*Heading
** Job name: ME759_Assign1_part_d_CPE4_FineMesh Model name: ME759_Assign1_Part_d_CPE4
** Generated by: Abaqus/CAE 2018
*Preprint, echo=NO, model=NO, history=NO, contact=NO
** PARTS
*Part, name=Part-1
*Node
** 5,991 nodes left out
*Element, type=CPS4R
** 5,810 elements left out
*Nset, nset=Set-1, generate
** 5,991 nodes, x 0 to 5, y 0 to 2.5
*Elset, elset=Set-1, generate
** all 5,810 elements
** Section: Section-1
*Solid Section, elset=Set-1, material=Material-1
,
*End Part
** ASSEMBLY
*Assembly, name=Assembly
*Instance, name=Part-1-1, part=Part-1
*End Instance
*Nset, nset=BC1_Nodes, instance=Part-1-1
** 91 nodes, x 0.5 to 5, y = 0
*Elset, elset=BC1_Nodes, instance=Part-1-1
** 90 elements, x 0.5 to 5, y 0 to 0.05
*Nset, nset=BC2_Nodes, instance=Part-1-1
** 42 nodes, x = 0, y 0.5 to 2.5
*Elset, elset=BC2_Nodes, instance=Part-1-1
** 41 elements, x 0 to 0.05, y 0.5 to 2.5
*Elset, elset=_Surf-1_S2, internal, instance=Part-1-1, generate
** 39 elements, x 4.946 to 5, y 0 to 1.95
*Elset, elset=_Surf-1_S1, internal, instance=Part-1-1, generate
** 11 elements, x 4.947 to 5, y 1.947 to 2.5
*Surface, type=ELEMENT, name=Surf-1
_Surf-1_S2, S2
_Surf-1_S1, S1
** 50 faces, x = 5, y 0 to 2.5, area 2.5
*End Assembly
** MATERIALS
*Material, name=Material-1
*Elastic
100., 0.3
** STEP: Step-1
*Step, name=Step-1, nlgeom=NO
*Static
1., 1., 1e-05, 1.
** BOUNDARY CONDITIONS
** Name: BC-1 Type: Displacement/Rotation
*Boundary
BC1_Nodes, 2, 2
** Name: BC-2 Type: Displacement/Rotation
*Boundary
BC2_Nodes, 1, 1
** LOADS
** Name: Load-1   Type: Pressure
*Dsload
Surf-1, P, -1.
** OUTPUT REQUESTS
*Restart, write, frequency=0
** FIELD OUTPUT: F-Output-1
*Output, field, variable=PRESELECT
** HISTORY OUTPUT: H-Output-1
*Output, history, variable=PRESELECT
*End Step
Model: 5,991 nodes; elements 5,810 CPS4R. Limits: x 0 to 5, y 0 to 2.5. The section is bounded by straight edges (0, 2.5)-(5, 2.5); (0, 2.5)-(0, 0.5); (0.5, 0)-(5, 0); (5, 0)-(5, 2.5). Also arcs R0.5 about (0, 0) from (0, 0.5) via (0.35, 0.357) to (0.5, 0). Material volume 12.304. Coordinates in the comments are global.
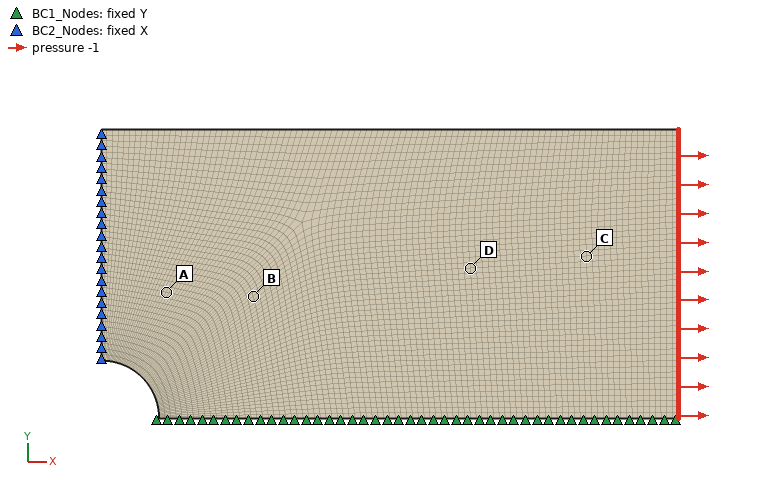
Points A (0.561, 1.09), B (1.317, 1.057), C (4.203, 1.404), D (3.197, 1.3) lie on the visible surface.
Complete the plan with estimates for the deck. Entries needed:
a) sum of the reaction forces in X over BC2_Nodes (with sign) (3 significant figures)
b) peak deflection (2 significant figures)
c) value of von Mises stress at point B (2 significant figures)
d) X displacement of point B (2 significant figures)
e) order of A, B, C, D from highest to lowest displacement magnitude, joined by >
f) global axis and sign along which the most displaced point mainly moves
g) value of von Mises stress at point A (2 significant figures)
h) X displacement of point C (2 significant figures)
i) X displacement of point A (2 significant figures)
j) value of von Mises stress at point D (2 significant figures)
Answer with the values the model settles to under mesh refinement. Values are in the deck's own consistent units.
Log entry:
-2.50
0.053
1.1
0.016
C > D > B > A
+X
1.2
0.044
0.0066
1.0
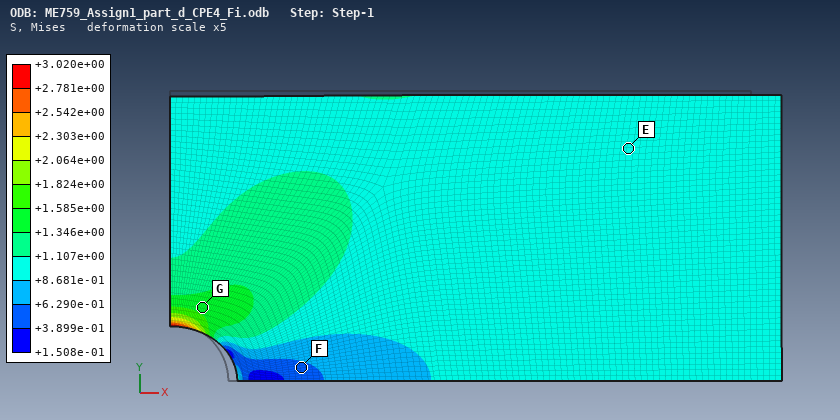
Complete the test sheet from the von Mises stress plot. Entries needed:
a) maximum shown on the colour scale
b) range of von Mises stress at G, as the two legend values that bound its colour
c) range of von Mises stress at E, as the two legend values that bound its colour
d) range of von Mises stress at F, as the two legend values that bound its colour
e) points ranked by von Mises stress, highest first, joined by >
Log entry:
+3.020e+00
+1.346e+00 to +1.585e+00
+8.681e-01 to +1.107e+00
+3.899e-01 to +6.290e-01
G > E > F
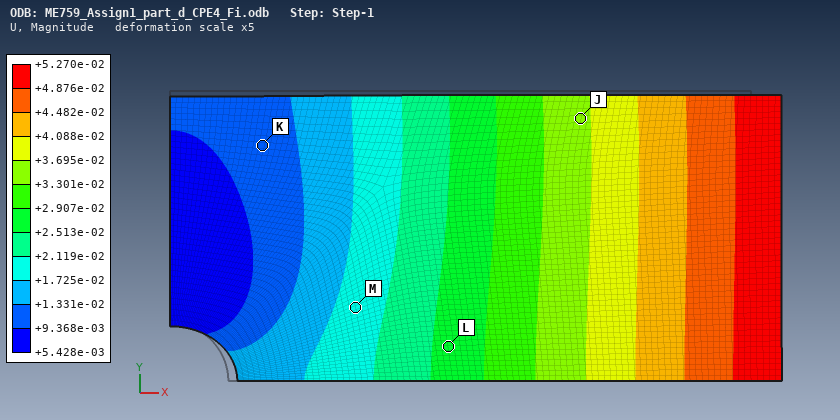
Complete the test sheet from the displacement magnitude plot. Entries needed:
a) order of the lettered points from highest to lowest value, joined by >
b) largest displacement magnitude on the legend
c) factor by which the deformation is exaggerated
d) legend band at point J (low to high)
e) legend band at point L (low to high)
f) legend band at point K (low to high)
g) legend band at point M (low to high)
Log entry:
J > L > M > K
+5.270e-02
5
+3.301e-02 to +3.695e-02
+2.513e-02 to +2.907e-02
+9.368e-03 to +1.331e-02
+1.725e-02 to +2.119e-02
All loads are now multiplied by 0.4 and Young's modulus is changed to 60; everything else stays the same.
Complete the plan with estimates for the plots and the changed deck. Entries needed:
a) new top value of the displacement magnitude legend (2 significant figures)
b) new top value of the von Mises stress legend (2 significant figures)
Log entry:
0.035
1.2
